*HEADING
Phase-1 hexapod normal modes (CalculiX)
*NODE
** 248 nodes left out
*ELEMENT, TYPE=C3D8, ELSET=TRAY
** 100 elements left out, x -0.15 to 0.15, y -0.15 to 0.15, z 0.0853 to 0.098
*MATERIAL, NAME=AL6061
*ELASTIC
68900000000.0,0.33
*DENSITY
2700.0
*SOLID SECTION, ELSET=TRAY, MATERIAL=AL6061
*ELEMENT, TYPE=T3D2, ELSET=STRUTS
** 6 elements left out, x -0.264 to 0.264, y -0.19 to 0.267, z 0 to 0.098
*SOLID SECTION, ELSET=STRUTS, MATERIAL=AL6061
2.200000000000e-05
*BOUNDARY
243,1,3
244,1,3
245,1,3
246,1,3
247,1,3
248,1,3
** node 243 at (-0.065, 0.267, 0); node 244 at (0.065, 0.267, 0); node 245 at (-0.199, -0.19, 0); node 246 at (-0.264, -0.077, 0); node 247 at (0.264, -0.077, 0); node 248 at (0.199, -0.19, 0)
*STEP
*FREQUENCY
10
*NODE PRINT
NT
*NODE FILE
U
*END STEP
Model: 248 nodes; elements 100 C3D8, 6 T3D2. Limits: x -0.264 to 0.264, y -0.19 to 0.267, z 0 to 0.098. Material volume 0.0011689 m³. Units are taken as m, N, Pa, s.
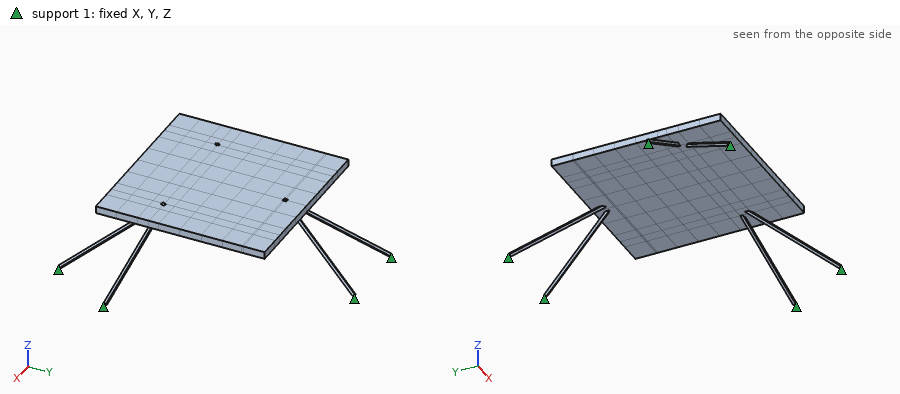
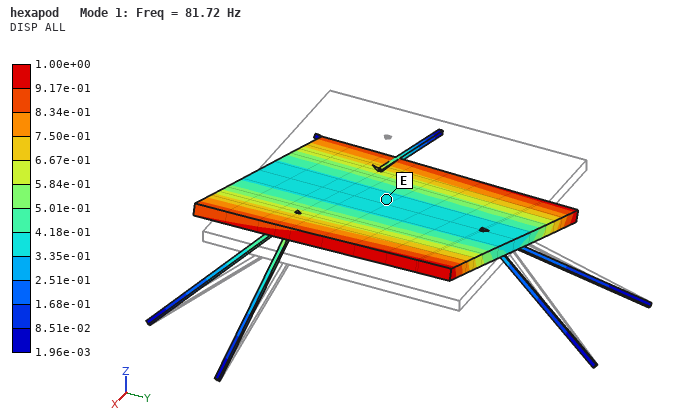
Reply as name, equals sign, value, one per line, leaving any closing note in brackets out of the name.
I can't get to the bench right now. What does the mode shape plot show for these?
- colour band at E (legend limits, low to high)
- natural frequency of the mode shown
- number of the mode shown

colour band at E = 3.35e-01 to 4.18e-01
natural frequency of the mode shown = 81.72 Hz
number of the mode shown = 1
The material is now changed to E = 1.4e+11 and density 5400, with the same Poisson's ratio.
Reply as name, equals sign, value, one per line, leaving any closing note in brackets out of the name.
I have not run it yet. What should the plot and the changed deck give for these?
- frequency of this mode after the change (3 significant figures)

frequency of this mode after the change = 82.4 Hz
